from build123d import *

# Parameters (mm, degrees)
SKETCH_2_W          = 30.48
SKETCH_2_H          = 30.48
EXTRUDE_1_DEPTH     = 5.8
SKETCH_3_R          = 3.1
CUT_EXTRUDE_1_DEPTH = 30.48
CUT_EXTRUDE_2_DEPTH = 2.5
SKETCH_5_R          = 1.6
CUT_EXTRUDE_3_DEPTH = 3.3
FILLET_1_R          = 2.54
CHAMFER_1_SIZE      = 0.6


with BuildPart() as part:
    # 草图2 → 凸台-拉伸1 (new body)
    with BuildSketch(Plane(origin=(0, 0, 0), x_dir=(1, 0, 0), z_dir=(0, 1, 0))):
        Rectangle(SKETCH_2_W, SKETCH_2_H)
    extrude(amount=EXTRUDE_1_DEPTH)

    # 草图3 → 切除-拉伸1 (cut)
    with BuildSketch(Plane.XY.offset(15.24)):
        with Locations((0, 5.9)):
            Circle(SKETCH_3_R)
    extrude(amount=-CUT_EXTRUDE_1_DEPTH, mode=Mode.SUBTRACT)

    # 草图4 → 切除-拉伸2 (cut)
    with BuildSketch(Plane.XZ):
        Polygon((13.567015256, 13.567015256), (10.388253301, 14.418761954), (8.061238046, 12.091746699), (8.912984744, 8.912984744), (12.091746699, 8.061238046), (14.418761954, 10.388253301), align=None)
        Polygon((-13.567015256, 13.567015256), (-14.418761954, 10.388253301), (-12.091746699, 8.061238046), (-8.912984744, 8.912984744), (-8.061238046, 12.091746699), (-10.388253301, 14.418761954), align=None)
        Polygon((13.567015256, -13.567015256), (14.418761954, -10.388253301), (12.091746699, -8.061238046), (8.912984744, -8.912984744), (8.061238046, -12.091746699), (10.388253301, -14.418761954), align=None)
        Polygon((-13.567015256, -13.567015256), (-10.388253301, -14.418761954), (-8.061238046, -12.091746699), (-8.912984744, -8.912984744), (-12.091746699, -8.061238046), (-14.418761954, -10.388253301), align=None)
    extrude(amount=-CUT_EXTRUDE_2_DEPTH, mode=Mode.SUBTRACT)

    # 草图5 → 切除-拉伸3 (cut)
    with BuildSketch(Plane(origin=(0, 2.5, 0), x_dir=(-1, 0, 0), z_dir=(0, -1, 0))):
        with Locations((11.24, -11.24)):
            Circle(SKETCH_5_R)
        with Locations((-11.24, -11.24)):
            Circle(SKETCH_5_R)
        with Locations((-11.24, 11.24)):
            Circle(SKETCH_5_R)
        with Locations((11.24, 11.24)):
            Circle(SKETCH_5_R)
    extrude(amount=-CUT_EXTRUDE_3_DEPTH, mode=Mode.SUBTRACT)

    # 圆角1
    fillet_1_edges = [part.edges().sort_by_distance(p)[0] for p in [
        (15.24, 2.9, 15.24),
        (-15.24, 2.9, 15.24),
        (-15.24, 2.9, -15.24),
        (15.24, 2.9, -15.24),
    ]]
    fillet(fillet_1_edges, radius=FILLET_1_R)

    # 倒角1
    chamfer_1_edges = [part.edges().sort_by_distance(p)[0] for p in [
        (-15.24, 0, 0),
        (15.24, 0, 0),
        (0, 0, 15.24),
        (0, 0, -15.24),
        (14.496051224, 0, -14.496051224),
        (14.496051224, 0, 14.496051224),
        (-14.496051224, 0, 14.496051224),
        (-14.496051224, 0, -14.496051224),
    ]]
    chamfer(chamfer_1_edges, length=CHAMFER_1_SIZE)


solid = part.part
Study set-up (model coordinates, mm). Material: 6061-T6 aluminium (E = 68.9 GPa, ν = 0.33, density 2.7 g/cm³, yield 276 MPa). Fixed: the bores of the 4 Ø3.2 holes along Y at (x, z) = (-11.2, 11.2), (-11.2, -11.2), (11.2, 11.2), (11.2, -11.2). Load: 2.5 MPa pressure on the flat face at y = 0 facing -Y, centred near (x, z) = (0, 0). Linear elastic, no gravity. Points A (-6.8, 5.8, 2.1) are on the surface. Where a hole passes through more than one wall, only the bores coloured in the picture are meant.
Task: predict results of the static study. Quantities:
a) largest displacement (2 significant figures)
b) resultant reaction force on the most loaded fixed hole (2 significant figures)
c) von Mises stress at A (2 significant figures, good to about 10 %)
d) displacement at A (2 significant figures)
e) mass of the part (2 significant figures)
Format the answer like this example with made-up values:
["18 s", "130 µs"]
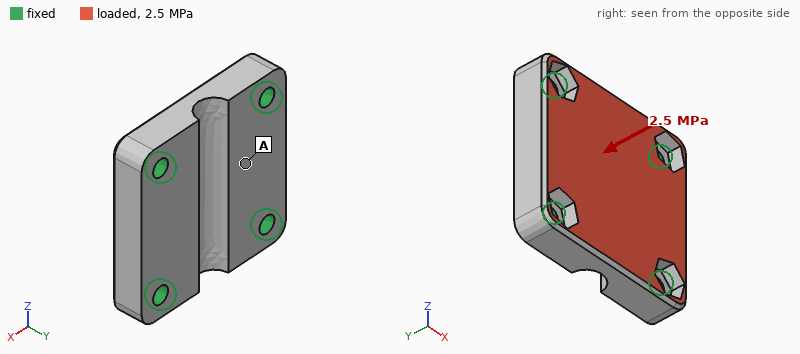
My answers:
["9.0 µm", "600 N", "10 MPa", "6.4 µm", "12 g"]
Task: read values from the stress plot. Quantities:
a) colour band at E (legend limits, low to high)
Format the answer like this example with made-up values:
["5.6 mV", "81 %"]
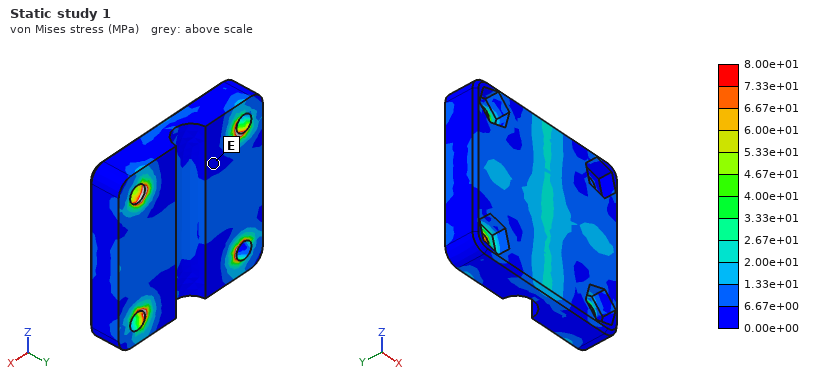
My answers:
["0.00e+00 to 6.67e+00 MPa"]
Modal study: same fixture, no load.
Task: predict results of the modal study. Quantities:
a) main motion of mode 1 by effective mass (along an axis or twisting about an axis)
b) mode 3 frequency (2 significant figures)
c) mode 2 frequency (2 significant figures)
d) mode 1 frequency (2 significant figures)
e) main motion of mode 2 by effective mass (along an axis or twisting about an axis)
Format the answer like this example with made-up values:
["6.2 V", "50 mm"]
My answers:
["along Y", "42 kHz", "40 kHz", "28 kHz", "twisting about Z"]
